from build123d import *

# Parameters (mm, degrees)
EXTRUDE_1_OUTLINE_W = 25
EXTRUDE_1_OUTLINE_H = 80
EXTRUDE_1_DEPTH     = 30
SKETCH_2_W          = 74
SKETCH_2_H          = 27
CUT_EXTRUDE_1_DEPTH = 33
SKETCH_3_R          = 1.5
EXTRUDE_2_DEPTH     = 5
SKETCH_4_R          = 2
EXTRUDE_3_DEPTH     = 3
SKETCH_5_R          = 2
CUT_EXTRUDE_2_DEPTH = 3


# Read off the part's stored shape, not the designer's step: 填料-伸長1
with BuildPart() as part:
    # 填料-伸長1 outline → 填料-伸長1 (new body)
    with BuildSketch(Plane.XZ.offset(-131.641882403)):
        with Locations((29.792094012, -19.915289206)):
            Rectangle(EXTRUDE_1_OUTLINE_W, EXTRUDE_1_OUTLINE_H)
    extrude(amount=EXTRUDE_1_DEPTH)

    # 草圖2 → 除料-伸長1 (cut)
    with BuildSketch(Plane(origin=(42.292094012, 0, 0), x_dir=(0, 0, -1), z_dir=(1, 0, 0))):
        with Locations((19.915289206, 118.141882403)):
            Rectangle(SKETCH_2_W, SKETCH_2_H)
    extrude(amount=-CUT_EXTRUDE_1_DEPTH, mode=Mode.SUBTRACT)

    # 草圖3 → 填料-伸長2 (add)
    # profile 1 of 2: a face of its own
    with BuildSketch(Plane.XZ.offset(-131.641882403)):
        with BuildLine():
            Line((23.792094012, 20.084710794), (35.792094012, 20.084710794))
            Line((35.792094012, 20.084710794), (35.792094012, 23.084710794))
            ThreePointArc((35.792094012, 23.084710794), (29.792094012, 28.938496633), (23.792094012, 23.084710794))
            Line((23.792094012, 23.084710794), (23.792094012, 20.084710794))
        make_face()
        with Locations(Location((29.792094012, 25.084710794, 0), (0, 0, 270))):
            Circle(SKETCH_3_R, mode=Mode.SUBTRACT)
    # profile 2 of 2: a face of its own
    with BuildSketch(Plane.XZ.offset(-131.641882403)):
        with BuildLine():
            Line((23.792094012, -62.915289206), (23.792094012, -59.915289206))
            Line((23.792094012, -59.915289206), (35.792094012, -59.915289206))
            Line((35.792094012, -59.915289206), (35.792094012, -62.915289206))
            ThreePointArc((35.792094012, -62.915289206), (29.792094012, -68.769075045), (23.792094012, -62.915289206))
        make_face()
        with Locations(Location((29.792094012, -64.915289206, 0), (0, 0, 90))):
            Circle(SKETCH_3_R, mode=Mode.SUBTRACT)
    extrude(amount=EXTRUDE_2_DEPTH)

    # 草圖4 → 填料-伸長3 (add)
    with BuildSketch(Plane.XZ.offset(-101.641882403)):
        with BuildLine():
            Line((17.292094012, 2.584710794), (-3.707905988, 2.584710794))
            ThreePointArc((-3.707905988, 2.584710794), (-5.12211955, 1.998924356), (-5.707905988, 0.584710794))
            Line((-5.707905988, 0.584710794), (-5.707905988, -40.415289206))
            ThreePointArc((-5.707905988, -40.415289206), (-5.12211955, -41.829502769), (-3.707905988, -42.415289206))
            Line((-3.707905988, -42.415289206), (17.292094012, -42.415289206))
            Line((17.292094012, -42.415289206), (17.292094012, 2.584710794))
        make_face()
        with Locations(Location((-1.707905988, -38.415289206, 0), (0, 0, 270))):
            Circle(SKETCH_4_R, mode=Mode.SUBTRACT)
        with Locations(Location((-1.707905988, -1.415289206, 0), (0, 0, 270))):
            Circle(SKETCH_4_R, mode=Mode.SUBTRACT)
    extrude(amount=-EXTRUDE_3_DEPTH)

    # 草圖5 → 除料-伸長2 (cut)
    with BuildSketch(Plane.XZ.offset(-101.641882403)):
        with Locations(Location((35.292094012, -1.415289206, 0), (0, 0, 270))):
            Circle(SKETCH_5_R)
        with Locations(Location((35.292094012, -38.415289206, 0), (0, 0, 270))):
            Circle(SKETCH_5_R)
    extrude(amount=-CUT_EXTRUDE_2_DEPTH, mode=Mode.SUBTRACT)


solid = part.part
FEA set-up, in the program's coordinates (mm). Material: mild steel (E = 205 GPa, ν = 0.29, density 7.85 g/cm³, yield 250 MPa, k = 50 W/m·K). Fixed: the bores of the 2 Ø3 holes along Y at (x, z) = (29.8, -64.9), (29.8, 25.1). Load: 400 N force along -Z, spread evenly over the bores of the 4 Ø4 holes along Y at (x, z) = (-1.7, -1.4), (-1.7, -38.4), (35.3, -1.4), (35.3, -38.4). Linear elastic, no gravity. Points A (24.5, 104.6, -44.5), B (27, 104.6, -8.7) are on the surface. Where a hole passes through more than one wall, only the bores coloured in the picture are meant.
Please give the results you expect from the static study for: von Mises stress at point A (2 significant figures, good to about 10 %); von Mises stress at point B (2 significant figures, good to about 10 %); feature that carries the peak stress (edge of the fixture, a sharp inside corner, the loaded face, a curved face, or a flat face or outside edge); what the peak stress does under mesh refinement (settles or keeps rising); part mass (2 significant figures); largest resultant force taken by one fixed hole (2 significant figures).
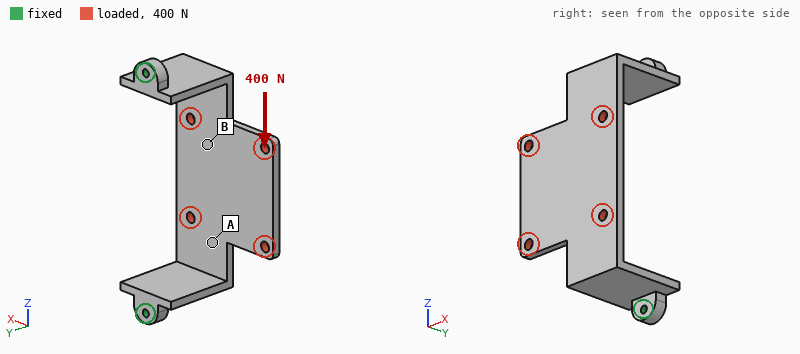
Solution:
37 MPa
12 MPa
edge of the fixture
keeps rising
110 g
220 N
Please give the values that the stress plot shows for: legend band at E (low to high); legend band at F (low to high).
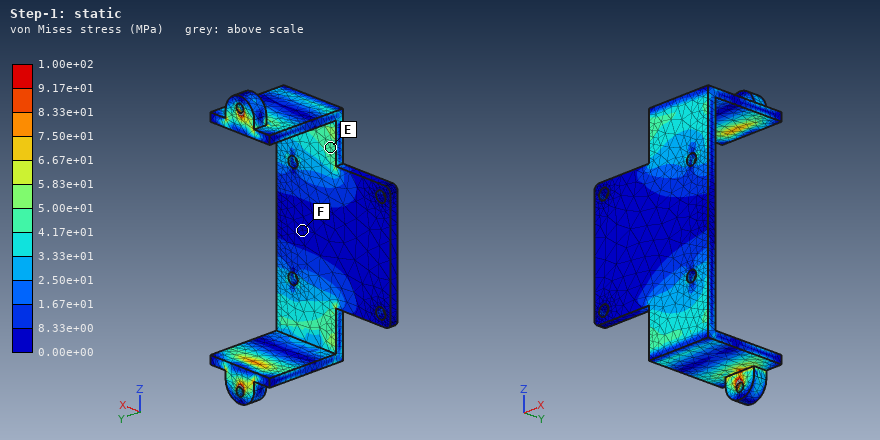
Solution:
4.17e+01 to 5.00e+01 MPa
0.00e+00 to 8.33e+00 MPa
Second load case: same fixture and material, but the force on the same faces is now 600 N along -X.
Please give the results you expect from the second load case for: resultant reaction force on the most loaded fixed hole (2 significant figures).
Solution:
300 N
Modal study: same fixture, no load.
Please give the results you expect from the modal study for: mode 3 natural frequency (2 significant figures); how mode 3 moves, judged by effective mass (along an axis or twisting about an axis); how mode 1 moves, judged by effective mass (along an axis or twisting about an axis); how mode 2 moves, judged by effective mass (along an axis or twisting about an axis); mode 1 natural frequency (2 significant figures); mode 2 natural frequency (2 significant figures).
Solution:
2000 Hz
along X
along Y
along Z
1200 Hz
1500 Hz
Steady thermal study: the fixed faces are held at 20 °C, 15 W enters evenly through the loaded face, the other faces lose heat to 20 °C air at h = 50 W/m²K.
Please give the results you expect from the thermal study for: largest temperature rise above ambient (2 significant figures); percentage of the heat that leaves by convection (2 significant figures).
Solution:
57 K
78 %
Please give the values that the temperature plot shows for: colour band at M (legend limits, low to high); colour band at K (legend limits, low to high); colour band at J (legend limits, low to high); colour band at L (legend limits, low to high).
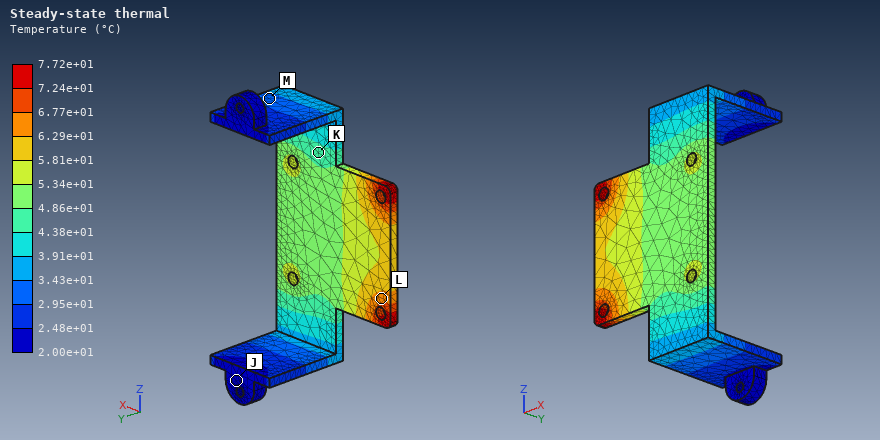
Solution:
2.95e+01 to 3.43e+01 °C
4.38e+01 to 4.86e+01 °C
2.00e+01 to 2.48e+01 °C
6.29e+01 to 6.77e+01 °C
